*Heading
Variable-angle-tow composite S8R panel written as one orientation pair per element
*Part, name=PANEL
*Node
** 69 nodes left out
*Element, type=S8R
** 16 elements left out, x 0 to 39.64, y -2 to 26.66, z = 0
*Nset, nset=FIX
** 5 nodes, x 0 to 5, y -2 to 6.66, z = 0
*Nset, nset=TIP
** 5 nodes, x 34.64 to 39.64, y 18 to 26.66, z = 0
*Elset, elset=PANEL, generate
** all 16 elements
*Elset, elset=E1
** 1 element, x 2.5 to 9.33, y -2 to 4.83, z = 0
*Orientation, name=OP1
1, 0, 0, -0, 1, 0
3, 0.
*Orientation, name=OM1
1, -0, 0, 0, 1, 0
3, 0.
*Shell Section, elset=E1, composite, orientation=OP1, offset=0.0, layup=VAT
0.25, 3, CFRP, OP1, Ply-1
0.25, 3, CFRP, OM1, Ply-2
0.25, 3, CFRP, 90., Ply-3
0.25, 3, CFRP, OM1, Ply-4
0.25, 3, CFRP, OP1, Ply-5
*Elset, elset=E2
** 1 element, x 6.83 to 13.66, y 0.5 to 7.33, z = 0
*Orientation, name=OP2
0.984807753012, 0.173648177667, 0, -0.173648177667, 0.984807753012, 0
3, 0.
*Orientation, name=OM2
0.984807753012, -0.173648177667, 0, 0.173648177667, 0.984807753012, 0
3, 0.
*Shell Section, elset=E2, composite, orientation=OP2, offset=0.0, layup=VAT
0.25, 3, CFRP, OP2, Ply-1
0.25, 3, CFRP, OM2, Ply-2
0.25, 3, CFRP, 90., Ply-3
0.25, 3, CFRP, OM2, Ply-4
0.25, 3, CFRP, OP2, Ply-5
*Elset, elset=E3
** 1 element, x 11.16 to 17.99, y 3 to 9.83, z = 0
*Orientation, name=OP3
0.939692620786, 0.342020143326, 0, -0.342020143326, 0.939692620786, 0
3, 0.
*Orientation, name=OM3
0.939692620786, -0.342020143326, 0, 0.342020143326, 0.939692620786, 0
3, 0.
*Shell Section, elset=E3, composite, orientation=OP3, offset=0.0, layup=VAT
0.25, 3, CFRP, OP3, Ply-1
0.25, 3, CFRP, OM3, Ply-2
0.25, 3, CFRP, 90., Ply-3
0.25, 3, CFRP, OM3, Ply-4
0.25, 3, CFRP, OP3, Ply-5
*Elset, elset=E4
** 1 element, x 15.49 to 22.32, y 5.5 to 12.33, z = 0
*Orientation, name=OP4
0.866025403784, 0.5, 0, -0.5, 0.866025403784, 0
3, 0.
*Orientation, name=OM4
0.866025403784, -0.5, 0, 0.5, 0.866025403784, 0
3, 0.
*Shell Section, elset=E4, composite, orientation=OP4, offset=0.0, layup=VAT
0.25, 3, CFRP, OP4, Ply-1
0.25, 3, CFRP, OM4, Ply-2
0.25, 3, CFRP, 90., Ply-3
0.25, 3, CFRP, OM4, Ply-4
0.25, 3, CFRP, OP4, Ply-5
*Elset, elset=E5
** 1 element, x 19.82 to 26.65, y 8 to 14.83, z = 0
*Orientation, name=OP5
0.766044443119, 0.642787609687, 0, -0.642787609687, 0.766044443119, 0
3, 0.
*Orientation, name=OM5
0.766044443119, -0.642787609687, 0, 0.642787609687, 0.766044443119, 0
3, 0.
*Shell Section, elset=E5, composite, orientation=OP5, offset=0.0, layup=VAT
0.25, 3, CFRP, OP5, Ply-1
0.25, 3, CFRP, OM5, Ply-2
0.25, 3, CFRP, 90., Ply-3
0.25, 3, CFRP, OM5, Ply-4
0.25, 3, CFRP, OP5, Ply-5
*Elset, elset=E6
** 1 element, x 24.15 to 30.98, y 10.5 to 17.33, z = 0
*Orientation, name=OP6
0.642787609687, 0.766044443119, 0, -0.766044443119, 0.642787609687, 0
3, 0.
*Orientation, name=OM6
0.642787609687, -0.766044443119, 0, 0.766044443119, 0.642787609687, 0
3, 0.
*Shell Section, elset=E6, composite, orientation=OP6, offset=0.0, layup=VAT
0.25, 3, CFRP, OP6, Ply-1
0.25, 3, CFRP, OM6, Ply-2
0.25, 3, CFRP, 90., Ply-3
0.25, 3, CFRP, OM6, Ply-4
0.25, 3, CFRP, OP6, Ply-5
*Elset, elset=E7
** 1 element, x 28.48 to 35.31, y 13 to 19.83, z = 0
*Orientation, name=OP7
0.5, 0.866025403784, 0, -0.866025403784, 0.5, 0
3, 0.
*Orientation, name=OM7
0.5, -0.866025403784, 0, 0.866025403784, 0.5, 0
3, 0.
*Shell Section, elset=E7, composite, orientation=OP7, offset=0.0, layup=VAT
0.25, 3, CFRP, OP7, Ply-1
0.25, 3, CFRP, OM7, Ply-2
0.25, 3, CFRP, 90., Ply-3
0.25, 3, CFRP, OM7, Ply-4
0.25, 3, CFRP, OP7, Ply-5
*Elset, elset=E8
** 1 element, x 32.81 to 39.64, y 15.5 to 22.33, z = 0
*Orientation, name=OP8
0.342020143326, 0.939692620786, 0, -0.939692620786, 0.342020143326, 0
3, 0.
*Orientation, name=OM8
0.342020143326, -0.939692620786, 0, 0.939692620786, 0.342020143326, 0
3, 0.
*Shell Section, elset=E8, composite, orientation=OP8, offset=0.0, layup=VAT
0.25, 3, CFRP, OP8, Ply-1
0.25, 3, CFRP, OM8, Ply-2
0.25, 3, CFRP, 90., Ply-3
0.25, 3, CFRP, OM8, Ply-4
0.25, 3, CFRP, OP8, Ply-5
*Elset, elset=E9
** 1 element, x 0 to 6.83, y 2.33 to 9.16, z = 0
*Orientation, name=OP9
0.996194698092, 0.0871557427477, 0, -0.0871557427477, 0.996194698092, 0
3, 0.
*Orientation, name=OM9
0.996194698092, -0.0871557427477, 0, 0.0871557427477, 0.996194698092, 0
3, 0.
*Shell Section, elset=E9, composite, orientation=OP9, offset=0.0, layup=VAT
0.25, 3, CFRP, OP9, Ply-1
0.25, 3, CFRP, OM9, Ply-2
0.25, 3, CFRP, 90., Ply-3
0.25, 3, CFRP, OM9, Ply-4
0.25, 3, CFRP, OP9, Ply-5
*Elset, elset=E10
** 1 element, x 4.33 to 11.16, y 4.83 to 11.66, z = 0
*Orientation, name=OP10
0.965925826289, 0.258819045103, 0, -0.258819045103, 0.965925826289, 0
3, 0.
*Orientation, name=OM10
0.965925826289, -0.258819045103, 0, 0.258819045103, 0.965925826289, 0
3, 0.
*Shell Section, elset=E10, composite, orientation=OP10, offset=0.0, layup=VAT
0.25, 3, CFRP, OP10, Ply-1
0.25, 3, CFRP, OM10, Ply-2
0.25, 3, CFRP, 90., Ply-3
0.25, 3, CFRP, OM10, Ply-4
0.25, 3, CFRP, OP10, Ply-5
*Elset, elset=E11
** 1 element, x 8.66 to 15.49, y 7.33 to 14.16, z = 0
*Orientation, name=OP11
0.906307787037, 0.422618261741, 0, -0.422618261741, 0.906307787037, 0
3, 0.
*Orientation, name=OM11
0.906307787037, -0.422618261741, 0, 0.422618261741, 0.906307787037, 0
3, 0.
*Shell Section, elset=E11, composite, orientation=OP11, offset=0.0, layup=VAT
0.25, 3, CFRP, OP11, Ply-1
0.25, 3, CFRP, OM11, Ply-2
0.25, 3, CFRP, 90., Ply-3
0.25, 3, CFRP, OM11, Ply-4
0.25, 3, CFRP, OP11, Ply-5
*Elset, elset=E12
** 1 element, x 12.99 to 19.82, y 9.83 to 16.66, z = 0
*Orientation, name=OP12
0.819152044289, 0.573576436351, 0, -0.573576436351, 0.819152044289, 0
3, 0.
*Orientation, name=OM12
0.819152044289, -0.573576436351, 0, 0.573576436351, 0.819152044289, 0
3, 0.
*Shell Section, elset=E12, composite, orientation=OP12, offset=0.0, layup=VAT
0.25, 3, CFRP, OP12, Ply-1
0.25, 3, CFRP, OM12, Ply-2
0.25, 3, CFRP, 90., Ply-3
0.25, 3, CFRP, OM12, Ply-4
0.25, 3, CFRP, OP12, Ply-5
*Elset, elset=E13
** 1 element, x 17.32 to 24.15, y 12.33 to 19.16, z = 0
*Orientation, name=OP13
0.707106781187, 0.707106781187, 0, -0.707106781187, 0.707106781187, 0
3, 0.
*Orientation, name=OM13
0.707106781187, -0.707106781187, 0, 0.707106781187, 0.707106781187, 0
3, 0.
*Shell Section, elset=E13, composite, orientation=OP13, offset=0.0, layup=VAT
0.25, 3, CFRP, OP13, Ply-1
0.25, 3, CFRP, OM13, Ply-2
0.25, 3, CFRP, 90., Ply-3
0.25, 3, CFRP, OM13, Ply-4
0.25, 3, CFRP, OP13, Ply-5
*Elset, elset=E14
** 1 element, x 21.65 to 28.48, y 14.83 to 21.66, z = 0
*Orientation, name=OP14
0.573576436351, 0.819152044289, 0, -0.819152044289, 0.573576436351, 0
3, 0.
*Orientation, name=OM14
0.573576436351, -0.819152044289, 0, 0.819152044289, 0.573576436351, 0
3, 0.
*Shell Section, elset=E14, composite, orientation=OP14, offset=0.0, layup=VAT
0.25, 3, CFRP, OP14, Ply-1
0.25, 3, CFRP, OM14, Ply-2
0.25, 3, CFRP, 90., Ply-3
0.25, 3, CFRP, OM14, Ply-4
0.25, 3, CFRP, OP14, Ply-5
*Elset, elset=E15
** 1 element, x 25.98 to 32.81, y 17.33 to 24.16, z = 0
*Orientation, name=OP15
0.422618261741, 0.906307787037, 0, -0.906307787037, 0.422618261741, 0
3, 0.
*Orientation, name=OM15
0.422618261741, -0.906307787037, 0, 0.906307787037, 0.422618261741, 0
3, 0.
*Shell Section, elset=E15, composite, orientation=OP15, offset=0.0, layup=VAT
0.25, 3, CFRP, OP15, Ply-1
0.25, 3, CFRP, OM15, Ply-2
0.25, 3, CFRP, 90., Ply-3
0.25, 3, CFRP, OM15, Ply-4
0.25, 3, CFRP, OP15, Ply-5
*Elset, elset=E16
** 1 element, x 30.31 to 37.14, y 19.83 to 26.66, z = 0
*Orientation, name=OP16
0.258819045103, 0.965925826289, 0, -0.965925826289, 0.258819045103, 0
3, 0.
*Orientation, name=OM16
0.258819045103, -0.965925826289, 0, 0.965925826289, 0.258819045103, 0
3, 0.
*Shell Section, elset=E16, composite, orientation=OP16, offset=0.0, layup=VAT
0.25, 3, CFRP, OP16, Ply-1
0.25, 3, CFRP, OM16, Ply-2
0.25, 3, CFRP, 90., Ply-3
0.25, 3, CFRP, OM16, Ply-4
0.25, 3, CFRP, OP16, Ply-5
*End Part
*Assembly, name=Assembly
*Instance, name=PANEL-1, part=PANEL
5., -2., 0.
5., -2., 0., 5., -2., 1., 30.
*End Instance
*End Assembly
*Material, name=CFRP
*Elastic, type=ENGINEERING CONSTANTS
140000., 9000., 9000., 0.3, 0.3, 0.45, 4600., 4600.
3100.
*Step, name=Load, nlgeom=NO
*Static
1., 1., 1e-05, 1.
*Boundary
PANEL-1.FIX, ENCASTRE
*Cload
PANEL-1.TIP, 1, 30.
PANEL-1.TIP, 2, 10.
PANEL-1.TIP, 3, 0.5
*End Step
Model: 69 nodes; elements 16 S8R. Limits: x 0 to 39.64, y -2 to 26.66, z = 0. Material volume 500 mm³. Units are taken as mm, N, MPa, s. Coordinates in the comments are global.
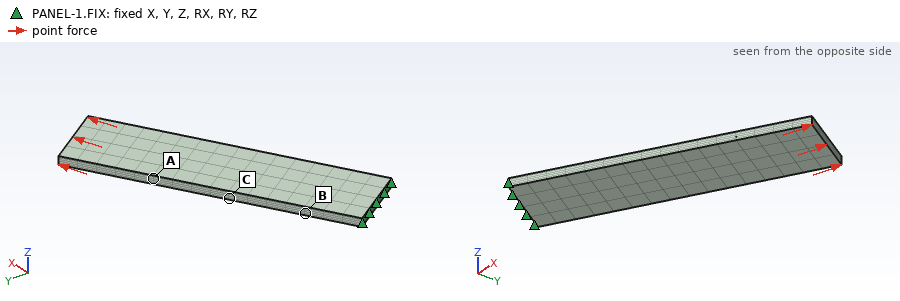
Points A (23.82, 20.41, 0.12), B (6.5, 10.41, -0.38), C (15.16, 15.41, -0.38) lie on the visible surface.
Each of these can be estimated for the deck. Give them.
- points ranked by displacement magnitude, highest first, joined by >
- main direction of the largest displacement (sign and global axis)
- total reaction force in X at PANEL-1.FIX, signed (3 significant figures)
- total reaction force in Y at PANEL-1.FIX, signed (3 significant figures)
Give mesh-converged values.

A > C > B
+Z
-150 N
-50.0 N
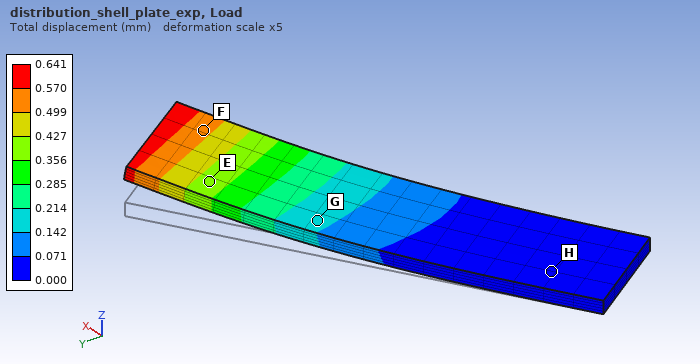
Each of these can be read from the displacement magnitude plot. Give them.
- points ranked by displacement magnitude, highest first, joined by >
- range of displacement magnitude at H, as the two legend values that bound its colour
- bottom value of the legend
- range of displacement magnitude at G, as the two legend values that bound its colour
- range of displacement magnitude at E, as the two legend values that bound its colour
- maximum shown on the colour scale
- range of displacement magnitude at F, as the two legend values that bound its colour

F > E > G > H
0.000 to 0.071 mm
0.000 mm
0.142 to 0.214 mm
0.356 to 0.427 mm
0.641 mm
0.499 to 0.570 mm
